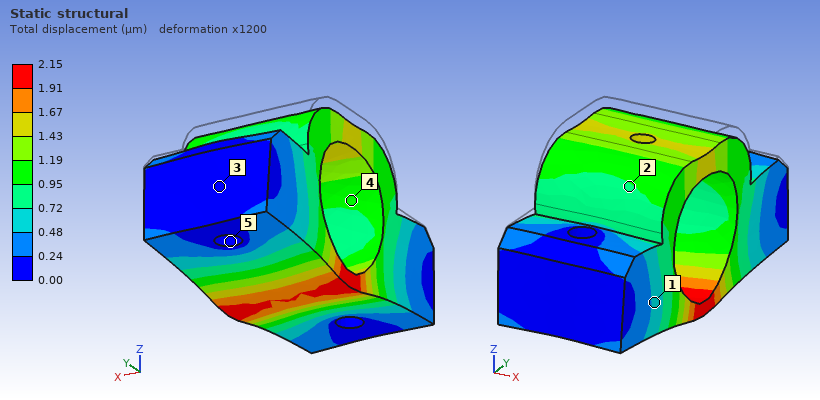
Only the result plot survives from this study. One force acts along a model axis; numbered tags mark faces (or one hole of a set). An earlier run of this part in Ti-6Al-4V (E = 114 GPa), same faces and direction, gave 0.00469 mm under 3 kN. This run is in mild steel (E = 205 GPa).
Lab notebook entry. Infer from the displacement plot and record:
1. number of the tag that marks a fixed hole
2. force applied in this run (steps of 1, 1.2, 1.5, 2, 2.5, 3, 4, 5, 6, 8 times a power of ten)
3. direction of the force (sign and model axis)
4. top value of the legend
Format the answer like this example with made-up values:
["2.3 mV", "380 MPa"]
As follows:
["5", "2.5 kN", "-Z", "2.15 µm"]
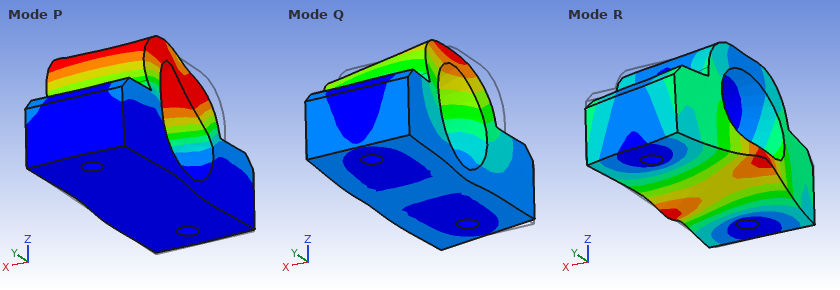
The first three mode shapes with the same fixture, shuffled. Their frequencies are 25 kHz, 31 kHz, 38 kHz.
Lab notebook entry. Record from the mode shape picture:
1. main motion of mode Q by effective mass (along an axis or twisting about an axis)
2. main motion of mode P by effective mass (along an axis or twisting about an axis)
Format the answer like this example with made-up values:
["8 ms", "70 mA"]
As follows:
["along X", "along Y"]
